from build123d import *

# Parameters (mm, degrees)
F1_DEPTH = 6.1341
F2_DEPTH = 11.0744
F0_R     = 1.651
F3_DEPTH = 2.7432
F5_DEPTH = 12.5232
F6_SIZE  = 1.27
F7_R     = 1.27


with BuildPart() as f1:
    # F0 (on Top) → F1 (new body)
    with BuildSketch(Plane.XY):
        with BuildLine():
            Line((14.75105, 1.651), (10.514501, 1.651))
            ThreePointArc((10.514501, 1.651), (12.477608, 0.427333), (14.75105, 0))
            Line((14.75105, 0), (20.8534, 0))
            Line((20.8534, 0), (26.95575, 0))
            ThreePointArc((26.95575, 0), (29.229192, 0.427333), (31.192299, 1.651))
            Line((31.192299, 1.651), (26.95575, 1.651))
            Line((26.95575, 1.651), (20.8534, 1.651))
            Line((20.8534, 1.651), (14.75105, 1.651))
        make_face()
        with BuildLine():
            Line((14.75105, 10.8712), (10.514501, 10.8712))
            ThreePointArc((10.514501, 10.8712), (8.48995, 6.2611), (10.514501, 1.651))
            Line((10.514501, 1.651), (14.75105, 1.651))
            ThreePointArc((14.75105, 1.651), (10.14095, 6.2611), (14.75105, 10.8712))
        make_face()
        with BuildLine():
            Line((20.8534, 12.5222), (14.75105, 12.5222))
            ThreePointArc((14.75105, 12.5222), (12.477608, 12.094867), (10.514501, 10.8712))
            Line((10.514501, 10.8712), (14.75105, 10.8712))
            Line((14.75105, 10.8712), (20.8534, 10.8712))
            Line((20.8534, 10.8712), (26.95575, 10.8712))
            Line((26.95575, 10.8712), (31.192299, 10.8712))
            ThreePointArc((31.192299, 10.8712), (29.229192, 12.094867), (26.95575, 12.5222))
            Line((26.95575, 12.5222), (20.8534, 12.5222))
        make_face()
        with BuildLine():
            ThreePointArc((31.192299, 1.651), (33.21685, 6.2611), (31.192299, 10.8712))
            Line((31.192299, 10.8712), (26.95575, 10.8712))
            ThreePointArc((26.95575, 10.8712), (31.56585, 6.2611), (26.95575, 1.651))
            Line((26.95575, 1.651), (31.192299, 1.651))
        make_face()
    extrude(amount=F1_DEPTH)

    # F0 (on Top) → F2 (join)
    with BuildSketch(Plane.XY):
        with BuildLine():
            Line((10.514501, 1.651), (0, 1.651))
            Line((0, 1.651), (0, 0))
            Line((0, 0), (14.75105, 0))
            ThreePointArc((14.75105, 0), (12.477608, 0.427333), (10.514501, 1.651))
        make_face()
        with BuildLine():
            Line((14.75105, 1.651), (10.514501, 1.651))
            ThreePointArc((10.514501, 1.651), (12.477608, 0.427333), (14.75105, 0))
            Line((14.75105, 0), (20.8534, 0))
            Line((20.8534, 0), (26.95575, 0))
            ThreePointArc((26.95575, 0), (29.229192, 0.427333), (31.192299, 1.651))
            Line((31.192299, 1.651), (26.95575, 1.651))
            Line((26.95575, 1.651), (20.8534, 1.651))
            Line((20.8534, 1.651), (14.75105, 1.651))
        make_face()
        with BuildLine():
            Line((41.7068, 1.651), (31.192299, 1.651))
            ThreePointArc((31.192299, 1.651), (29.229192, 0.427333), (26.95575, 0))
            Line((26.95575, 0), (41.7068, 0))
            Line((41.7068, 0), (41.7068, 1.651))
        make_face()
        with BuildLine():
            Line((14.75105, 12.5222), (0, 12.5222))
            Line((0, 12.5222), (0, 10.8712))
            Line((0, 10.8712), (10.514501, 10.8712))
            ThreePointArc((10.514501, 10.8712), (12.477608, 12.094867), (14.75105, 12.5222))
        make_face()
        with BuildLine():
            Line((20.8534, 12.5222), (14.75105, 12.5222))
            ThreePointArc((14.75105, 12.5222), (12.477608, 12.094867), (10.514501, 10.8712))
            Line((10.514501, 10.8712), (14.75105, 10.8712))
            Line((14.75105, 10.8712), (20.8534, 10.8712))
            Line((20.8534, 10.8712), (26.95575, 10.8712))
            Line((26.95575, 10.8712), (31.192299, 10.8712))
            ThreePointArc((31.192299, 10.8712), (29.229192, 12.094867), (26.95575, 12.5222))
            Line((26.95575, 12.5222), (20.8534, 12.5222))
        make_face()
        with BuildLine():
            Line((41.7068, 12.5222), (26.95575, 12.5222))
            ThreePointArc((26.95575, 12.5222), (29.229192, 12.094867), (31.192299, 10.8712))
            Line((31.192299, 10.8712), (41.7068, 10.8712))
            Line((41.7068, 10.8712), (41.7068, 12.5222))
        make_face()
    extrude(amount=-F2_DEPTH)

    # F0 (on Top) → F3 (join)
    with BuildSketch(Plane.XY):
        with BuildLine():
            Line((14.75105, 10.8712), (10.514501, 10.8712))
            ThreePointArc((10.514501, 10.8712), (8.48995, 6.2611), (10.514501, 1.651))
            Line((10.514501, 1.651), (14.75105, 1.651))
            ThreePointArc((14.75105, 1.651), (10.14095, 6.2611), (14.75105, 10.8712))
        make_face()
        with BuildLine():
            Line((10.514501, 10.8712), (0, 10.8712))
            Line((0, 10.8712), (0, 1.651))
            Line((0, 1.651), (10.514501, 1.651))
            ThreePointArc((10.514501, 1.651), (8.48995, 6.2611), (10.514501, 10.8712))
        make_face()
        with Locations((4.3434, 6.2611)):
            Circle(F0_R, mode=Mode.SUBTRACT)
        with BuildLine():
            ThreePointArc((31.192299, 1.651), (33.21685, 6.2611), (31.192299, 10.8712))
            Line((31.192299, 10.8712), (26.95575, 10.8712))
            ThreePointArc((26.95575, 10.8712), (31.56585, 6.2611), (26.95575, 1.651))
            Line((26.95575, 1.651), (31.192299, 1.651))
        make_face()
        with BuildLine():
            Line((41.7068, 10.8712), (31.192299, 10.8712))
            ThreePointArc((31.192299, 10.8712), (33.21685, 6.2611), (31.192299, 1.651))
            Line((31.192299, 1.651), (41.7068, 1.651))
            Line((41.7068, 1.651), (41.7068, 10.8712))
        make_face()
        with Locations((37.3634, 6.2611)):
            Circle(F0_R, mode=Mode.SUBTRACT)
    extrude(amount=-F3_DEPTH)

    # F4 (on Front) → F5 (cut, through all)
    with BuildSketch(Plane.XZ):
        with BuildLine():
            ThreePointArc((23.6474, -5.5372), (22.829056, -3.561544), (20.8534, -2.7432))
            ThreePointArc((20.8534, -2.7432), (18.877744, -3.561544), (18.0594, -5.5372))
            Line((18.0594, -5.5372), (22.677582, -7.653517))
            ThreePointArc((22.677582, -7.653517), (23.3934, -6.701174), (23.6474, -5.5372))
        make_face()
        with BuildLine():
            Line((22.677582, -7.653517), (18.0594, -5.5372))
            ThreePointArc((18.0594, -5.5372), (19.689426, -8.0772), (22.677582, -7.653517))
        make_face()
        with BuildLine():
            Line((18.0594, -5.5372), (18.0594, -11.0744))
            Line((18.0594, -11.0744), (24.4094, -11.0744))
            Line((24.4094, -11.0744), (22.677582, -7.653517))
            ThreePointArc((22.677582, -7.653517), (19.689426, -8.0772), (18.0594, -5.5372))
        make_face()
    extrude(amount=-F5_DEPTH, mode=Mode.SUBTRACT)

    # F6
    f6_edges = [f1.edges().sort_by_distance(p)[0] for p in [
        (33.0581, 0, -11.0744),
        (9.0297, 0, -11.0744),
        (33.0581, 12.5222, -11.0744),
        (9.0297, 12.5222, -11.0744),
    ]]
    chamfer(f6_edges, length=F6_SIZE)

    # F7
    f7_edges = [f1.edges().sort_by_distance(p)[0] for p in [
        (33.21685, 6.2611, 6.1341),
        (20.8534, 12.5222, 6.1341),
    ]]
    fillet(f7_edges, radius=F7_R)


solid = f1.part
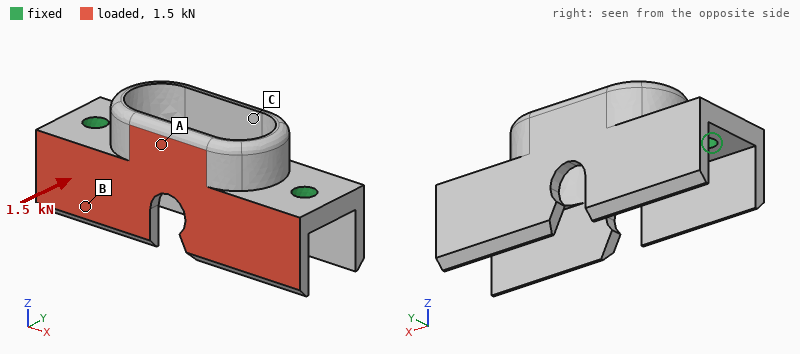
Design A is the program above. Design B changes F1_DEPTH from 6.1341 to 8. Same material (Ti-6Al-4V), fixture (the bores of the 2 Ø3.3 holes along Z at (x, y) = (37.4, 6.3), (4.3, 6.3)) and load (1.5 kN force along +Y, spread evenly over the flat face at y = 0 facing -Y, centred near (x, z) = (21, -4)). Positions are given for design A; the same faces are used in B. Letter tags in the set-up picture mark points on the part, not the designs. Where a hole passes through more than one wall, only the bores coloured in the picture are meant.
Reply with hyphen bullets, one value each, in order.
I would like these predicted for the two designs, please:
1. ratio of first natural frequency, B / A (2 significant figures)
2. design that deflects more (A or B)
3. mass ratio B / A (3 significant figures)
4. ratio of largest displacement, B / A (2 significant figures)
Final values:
- 0.95
- A
- 1.07
- 0.91
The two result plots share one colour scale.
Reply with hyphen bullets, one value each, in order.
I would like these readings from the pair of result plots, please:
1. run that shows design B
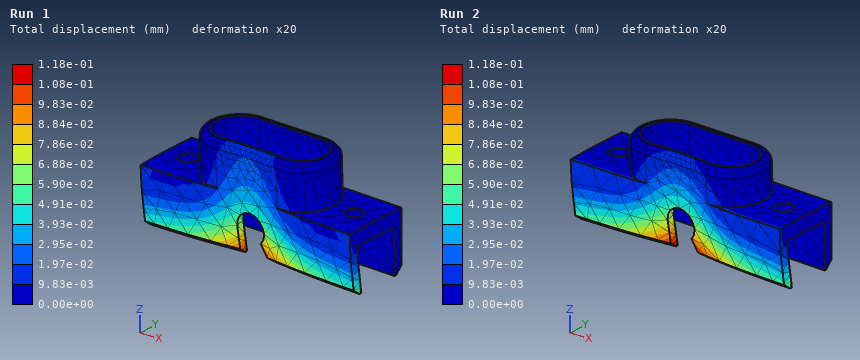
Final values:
- Run 1
